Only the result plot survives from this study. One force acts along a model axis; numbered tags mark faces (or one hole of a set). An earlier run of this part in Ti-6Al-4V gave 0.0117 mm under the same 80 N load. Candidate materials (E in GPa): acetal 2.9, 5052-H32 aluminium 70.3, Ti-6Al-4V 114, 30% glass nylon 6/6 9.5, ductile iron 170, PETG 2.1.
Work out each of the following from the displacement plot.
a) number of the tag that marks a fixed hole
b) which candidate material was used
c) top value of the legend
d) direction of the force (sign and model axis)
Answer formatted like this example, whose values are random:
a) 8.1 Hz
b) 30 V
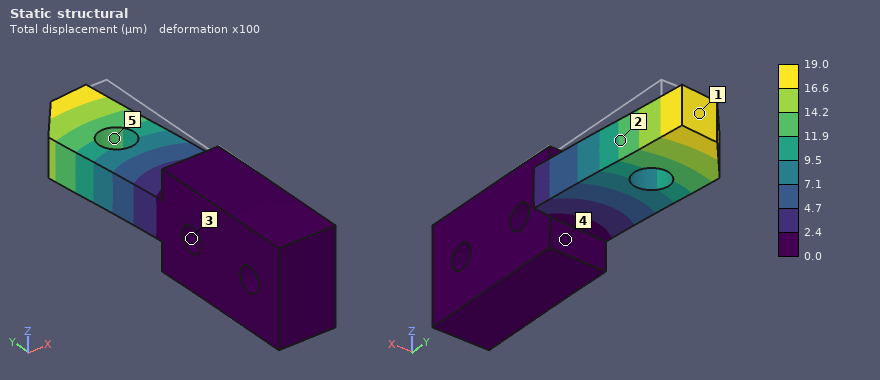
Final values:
a) 3
b) 5052-H32 aluminium
c) 19.0 µm
d) -X
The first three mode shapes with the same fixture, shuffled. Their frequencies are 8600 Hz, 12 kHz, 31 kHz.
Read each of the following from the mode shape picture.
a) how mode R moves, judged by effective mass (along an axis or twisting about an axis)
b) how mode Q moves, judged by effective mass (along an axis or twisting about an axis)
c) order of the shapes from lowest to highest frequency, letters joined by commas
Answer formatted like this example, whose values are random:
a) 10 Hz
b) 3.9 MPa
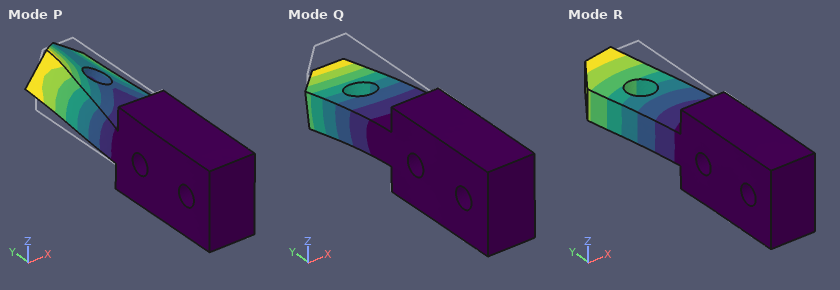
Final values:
a) along X
b) along Z
c) Q, R, P
